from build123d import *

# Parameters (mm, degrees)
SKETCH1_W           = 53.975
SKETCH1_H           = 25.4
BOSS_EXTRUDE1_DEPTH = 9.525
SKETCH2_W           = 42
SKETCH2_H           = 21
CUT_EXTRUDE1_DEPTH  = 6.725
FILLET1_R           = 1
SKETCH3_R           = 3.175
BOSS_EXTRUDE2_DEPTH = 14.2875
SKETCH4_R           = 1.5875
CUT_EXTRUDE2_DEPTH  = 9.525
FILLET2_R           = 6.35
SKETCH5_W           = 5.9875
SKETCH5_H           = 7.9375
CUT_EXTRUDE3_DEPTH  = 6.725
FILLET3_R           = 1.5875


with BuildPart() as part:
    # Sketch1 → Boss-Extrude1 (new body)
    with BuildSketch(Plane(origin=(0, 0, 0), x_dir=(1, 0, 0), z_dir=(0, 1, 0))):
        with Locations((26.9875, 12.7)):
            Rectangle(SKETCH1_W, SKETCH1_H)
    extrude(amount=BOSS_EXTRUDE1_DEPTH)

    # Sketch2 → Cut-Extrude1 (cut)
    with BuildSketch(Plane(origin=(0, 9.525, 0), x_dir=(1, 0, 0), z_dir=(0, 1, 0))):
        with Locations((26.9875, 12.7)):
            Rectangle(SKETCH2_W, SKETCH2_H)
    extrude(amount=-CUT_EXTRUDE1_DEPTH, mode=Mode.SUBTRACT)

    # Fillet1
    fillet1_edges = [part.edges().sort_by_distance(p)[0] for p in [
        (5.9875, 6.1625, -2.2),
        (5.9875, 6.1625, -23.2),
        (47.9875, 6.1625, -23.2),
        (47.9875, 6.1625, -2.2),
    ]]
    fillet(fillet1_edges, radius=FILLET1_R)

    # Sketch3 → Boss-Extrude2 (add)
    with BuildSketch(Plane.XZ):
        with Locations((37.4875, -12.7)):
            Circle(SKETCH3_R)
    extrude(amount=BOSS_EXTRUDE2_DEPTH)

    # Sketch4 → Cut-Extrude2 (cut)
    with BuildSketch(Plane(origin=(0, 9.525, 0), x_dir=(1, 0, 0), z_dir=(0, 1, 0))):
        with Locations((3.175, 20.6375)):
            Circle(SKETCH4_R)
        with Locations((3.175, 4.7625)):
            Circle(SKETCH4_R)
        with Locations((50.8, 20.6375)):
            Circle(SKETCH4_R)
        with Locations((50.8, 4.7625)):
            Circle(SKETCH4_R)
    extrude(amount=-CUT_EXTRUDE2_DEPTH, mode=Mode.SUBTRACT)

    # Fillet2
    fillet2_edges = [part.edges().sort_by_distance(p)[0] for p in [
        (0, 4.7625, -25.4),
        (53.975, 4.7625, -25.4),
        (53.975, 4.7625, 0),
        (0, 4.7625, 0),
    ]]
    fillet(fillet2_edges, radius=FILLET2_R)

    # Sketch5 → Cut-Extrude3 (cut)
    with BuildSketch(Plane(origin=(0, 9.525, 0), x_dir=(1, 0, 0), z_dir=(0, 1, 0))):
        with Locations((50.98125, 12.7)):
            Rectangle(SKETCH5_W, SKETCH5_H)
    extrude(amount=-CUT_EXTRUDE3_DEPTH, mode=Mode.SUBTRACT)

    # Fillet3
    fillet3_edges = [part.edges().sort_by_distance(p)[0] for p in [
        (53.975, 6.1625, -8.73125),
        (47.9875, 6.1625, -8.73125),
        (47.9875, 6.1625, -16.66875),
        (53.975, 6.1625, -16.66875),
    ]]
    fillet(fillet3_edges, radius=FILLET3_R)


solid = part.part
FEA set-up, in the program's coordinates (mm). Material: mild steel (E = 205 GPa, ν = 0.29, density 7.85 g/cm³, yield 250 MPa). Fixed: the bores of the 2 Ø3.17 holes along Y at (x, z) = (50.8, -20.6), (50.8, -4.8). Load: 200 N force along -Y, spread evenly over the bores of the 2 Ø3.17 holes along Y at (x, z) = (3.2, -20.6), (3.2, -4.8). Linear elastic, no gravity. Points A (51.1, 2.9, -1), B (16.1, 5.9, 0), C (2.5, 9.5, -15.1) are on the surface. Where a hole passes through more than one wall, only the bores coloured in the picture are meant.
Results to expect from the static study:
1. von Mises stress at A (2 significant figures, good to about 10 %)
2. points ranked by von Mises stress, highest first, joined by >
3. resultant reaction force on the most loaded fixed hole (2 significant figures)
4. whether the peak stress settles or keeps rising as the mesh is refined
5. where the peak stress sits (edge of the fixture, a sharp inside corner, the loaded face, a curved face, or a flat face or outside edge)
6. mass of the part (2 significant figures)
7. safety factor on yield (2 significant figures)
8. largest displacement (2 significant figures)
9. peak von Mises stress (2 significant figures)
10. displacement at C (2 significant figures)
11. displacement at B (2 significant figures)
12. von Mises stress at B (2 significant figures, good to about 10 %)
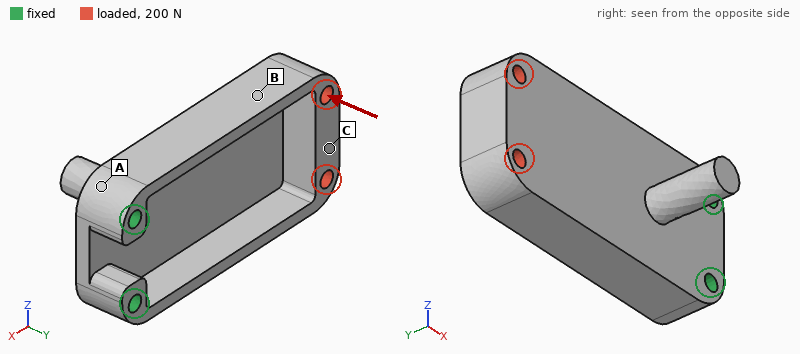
30 MPa
A > B > C
140 N
settles
a curved face
52 g
1.5
73 µm
170 MPa
68 µm
40 µm
16 MPa
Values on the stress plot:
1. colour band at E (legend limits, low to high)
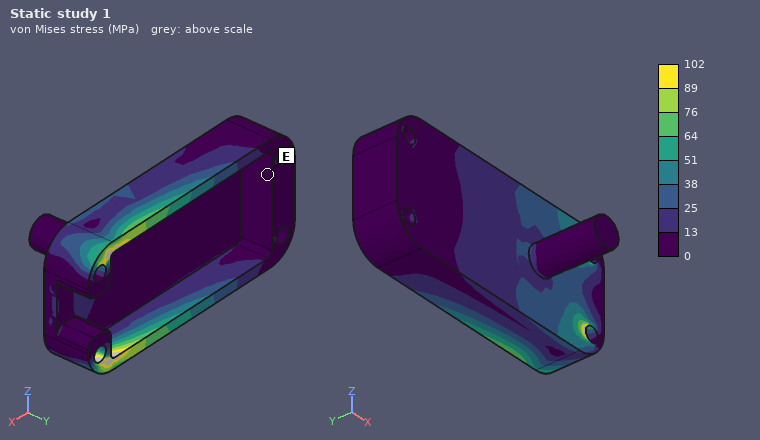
0 to 13 MPa
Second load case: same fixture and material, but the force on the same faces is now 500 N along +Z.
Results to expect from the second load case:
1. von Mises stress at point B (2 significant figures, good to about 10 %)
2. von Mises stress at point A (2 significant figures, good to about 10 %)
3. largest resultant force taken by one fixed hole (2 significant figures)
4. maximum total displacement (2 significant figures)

30 MPa
33 MPa
1.3 kN
51 µm
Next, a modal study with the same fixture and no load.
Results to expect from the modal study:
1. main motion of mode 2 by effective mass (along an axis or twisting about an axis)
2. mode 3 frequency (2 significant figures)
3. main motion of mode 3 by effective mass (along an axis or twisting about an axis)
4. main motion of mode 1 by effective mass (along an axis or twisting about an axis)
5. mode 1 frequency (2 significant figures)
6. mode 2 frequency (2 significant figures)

along Z
7300 Hz
along Z
along Y
2200 Hz
3900 Hz
